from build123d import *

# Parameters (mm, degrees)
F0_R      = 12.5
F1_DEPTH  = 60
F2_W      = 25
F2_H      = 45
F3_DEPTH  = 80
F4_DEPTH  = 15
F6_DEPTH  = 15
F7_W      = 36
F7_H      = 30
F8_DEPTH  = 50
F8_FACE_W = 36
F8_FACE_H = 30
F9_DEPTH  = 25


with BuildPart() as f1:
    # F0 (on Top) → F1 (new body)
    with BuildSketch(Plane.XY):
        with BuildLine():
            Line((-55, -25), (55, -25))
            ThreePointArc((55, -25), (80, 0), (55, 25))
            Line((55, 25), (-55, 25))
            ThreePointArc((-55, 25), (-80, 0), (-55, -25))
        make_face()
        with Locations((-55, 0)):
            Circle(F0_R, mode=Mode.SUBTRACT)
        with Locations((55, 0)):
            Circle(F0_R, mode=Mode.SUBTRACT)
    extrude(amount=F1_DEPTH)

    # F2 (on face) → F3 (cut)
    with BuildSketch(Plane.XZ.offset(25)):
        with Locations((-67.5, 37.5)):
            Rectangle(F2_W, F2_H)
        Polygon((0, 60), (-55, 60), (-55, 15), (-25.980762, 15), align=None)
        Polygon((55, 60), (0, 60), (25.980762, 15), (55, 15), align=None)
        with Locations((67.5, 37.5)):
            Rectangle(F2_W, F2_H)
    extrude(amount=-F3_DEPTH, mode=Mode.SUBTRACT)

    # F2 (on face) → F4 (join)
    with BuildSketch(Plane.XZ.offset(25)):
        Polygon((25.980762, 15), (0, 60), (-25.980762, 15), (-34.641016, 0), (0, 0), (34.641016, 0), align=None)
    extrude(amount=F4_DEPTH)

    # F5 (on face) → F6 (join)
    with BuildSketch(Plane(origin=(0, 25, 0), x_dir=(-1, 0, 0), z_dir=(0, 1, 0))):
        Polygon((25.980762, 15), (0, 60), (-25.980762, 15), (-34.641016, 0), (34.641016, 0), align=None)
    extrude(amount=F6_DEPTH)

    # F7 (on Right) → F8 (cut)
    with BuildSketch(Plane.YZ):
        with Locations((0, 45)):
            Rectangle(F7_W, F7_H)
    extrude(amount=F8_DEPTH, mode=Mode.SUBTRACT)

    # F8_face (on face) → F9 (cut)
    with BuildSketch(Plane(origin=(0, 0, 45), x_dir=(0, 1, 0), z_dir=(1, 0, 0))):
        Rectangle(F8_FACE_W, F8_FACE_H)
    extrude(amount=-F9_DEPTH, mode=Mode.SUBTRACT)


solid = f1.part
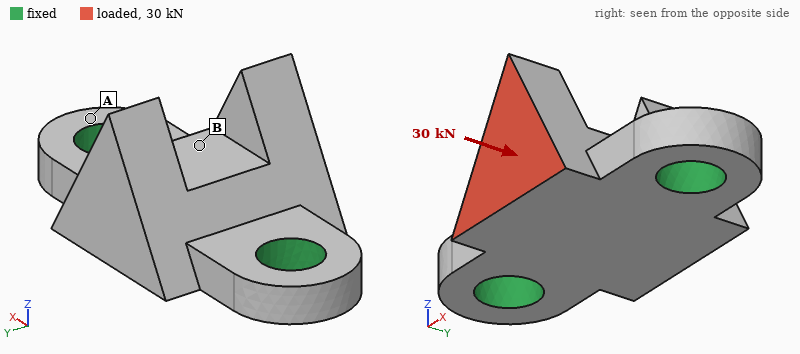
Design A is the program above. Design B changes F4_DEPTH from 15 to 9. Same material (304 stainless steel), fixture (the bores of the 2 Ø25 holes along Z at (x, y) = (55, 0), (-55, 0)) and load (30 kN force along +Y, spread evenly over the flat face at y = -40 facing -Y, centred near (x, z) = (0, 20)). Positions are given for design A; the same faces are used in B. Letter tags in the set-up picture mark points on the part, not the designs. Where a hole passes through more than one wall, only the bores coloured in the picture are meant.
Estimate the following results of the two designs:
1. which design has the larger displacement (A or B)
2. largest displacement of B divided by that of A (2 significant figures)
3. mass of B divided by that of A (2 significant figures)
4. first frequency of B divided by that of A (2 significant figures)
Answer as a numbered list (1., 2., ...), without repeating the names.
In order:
1. B
2. 1.1
3. 0.94
4. 1.1
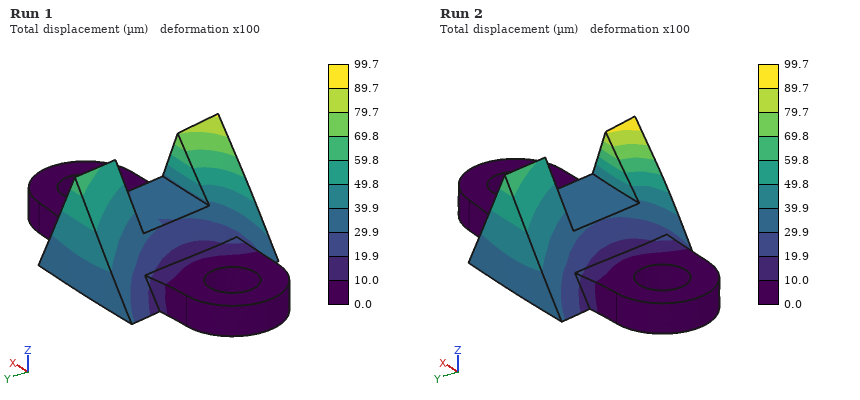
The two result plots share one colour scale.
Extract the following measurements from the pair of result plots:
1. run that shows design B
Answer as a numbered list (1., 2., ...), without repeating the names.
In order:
1. Run 2
